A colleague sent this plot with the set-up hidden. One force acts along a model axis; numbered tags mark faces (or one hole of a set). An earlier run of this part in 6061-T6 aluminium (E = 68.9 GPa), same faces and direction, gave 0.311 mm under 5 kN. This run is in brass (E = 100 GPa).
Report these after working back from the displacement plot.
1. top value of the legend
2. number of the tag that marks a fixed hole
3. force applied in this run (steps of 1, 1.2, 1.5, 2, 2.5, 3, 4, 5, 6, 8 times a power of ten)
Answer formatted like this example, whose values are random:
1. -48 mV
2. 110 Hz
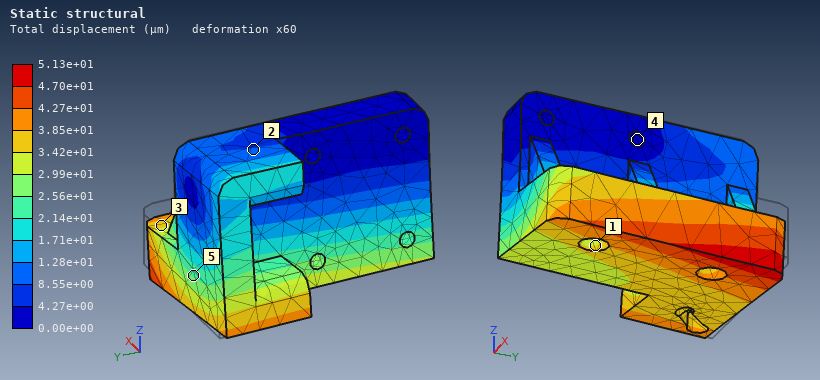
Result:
1. 5.13e+01 µm
2. 4
3. 1.2 kN
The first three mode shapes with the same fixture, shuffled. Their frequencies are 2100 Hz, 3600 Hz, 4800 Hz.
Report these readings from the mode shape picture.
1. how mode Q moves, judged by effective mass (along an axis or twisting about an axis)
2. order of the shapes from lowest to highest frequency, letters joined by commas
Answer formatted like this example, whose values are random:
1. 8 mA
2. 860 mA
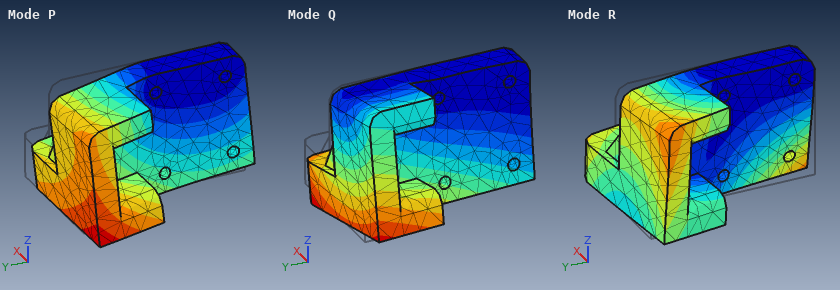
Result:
1. along X
2. Q, R, P
